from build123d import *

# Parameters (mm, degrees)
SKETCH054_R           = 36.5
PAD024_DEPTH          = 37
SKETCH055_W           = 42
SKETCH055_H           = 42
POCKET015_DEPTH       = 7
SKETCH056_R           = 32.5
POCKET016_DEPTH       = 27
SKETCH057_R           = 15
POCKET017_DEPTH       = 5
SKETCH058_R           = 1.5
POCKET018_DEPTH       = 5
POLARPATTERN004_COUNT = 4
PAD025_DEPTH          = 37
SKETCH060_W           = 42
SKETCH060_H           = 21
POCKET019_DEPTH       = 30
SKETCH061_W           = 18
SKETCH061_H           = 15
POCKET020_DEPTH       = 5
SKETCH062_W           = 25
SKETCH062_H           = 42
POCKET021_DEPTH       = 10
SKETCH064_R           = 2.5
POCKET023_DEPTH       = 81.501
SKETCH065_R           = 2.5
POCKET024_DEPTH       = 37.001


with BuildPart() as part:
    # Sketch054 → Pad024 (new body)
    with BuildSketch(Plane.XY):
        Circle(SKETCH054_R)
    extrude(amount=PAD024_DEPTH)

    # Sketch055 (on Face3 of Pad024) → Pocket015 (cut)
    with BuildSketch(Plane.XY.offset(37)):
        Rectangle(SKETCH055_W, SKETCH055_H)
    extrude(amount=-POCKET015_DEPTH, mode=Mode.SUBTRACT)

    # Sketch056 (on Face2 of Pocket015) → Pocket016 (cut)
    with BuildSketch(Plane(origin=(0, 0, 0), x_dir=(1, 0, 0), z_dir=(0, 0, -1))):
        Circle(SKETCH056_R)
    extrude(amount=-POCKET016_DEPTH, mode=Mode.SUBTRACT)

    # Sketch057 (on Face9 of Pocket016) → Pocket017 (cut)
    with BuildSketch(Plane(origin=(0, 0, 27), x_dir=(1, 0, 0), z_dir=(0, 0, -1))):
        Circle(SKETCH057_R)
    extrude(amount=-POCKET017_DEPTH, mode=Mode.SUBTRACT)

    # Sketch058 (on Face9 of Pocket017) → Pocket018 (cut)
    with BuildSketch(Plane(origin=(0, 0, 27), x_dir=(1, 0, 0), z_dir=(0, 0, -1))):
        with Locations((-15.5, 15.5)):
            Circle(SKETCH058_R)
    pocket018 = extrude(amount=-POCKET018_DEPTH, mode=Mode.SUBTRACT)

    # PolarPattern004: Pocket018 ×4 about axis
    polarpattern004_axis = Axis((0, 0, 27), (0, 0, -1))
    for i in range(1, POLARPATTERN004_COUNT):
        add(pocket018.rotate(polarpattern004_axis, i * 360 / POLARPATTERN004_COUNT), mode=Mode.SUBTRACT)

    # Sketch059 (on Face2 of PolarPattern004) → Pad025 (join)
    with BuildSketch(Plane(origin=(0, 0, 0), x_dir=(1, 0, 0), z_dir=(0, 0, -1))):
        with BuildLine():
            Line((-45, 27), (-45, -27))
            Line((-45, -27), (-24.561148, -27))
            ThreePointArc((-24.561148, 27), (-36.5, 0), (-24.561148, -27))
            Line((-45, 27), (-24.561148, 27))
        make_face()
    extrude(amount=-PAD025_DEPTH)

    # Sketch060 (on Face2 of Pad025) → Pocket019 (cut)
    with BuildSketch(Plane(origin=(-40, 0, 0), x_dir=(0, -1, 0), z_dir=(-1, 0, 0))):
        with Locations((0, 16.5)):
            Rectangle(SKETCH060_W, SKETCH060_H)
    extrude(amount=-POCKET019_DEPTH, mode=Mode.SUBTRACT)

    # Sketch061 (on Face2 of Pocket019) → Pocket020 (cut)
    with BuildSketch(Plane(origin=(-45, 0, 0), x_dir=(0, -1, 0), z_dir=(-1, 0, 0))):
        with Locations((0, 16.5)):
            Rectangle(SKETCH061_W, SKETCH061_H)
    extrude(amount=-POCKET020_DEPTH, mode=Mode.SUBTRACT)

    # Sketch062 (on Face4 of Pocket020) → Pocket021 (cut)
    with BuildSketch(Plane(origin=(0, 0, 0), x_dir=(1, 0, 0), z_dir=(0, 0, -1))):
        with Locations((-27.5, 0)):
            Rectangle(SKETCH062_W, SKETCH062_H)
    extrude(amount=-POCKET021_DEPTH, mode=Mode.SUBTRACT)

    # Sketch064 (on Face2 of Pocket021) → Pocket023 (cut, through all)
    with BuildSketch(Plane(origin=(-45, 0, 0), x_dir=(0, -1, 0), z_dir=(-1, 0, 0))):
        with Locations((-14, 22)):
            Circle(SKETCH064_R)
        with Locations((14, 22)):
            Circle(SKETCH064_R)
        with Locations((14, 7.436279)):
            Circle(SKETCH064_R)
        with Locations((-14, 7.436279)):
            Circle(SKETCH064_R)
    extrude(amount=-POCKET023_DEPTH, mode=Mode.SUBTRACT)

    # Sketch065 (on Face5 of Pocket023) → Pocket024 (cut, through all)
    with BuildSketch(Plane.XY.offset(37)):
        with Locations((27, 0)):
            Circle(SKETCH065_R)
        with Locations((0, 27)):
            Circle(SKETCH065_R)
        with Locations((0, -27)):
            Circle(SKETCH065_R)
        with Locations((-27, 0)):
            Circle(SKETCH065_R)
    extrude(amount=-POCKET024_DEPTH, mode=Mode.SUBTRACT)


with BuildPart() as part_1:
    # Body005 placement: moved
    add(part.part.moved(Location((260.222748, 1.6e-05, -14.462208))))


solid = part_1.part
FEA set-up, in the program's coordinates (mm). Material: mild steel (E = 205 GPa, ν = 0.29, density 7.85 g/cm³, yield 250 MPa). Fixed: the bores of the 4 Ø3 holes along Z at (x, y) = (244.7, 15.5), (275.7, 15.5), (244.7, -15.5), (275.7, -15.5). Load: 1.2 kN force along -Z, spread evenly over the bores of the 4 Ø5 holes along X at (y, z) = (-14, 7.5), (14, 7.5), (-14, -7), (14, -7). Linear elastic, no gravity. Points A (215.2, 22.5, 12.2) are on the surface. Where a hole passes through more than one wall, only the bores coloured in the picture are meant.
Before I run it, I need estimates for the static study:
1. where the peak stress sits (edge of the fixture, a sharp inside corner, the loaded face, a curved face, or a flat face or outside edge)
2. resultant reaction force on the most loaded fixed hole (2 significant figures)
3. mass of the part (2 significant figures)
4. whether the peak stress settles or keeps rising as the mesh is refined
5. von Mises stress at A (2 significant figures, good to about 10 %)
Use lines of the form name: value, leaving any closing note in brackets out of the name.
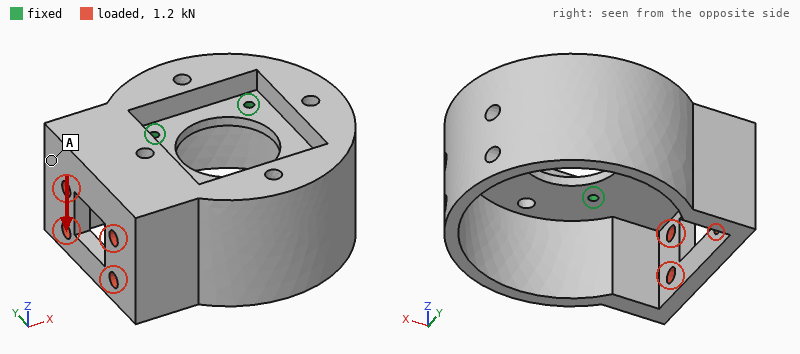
where the peak stress sits: edge of the fixture
resultant reaction force on the most loaded fixed hole: 1.1 kN
mass of the part: 480 g
whether the peak stress settles or keeps rising as the mesh is refined: keeps rising
von Mises stress at A: 7.2 MPa
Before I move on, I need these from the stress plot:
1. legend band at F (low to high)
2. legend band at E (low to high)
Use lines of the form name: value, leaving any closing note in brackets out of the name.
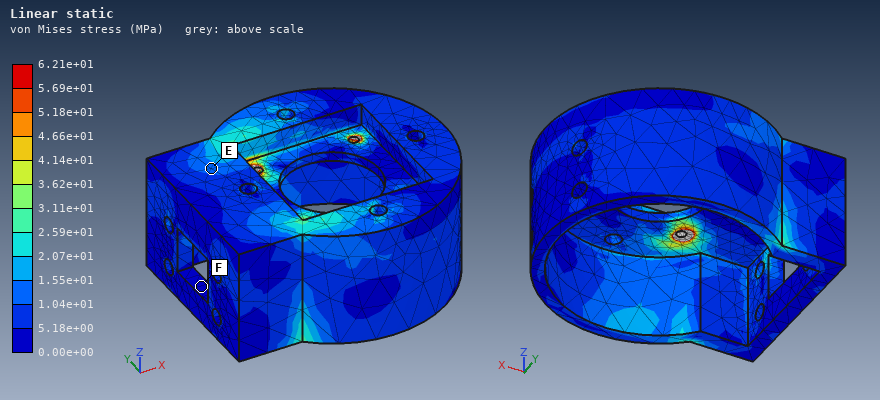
legend band at F: 0.00e+00 to 5.18e+00 MPa
legend band at E: 1.04e+01 to 1.55e+01 MPa
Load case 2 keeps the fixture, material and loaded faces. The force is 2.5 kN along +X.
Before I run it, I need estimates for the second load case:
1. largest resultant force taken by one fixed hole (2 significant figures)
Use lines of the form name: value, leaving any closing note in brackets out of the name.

largest resultant force taken by one fixed hole: 1.1 kN
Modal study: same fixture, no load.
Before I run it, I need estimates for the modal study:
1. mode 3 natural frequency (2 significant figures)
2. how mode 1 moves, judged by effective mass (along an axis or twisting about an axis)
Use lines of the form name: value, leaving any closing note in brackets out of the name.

mode 3 natural frequency: 4300 Hz
how mode 1 moves, judged by effective mass: along Z
